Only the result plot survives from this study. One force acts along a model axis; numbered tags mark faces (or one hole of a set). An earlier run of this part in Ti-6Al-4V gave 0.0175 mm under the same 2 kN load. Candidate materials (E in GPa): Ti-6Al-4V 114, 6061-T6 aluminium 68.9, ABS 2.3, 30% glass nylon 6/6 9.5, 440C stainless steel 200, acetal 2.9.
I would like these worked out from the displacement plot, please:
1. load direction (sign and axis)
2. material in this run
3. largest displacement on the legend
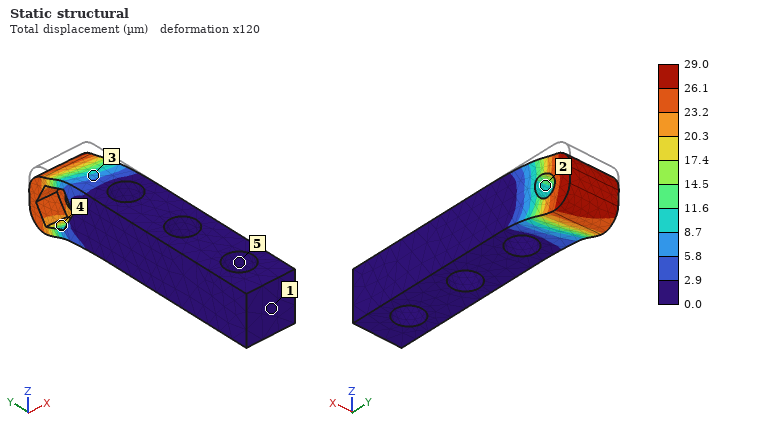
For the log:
-Z
6061-T6 aluminium
29.0 µm
